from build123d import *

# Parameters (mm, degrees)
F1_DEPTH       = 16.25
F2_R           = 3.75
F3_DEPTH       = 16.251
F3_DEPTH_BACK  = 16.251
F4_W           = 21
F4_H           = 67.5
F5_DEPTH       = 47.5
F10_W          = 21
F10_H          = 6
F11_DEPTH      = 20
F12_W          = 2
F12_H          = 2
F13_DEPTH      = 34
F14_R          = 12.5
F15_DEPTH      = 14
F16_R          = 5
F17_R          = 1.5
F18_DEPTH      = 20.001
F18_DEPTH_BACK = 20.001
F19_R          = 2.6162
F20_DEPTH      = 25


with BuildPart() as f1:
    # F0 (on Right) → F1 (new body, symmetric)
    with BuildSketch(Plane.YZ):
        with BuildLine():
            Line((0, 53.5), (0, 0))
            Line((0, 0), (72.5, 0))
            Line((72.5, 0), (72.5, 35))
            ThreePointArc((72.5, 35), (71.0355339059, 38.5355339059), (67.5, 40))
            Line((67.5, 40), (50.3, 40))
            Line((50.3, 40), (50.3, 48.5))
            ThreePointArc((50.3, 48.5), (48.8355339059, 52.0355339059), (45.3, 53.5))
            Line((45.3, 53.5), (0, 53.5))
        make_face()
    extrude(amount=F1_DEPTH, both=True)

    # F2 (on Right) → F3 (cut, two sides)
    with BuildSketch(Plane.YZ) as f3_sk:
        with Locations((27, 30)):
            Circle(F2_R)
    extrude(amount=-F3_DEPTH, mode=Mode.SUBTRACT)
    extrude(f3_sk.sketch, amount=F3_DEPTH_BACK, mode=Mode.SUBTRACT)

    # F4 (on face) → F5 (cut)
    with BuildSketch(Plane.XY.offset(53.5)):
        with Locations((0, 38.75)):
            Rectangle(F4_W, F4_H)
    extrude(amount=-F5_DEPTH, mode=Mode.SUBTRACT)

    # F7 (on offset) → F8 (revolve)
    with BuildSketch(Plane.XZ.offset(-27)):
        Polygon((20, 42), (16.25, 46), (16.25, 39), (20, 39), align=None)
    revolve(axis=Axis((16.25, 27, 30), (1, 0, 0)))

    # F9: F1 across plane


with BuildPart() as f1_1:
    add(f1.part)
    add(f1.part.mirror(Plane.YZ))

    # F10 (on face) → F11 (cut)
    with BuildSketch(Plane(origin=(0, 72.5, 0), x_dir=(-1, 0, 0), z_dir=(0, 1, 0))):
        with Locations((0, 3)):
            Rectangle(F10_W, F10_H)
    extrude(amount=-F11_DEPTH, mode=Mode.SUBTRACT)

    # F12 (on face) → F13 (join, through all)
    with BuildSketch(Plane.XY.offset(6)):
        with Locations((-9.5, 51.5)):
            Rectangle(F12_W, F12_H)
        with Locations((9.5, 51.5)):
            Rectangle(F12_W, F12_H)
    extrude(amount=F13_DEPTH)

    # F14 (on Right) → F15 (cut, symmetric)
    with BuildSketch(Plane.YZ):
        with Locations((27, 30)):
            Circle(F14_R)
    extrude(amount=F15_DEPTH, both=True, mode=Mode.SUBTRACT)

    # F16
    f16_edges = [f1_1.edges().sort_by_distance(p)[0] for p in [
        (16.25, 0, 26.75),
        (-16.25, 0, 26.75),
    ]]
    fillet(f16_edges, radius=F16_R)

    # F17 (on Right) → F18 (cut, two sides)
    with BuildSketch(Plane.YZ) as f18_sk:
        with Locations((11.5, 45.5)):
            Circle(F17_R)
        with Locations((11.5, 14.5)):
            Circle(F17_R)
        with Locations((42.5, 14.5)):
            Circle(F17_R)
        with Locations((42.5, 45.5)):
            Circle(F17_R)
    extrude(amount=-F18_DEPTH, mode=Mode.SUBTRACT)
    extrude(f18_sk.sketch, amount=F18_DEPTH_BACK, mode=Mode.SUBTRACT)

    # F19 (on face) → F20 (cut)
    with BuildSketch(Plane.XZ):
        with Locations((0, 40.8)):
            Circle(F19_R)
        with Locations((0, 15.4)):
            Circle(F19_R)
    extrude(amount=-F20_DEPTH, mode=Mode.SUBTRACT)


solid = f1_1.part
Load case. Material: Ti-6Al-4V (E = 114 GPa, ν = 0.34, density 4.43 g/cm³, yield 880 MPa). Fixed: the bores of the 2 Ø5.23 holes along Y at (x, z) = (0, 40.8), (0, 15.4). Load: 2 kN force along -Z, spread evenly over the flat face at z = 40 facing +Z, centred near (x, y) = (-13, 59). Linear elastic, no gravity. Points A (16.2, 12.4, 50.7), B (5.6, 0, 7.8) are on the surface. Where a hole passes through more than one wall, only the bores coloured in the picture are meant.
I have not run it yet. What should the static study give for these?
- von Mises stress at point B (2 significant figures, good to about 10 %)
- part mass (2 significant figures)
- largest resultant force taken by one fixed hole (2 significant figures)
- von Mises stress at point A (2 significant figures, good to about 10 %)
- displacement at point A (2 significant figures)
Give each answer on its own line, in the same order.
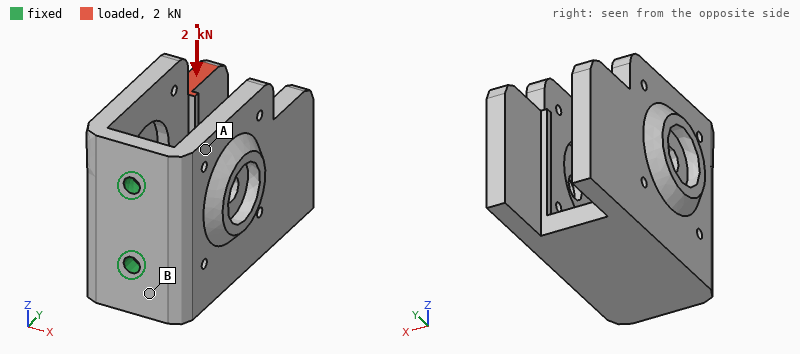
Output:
59 MPa
230 g
3.8 kN
18 MPa
0.042 mm
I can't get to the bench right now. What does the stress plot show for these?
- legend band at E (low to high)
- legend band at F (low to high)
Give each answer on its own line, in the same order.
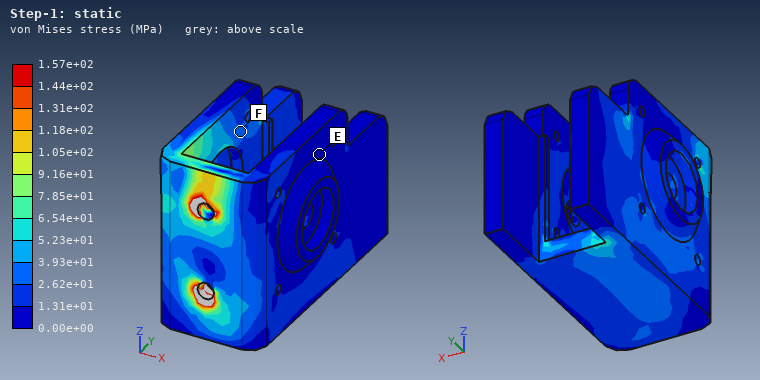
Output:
0.00e+00 to 1.31e+01 MPa
2.62e+01 to 3.93e+01 MPa
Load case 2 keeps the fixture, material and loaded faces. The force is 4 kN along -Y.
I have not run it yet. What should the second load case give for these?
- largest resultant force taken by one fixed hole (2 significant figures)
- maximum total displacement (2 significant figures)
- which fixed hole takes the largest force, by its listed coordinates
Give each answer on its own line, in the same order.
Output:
3.5 kN
0.19 mm
(0, 40.8)
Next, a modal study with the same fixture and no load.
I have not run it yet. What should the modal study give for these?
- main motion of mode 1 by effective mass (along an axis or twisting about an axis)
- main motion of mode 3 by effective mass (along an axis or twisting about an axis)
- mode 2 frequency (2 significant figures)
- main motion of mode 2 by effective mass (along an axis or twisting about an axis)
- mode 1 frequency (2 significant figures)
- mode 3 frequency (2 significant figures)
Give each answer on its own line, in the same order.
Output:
along X
along Z
2100 Hz
along Z
980 Hz
2700 Hz
